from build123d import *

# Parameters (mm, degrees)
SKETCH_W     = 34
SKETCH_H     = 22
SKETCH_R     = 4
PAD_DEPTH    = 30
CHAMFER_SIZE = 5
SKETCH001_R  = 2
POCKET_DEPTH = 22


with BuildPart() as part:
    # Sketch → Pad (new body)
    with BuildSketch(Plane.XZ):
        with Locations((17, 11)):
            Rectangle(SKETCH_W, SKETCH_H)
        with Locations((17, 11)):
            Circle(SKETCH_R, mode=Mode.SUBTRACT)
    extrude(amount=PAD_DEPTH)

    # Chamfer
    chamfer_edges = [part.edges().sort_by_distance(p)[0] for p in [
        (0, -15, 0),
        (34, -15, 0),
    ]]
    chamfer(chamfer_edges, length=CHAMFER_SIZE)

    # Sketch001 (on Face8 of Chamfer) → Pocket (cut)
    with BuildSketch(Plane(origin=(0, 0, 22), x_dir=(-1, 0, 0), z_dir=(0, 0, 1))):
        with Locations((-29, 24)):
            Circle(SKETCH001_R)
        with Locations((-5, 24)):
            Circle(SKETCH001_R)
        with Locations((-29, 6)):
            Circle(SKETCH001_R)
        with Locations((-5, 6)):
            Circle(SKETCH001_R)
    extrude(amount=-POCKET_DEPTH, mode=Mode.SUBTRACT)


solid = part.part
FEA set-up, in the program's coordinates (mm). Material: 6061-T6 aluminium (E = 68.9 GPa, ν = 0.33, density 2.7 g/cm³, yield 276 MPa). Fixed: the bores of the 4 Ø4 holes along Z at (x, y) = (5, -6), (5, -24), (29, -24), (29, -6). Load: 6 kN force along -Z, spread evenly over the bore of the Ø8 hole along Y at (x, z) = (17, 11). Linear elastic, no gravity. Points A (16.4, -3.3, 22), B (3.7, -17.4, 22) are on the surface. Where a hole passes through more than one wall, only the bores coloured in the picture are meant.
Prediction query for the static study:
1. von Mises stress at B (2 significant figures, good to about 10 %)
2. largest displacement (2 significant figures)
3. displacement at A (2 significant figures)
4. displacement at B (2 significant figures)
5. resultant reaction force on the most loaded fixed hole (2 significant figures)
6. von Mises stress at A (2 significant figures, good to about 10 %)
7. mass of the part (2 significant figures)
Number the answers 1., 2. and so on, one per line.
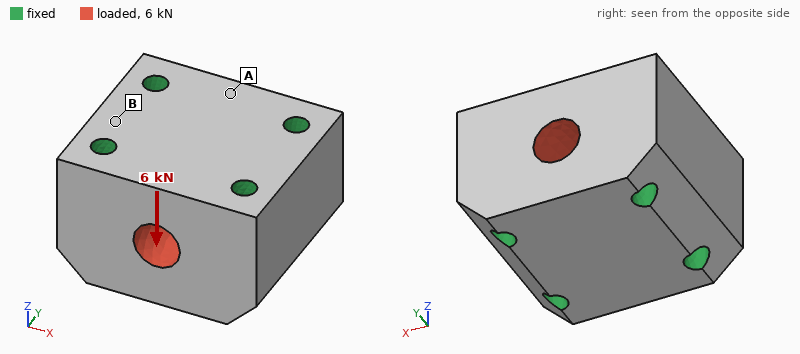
1. 3.1 MPa
2. 2.6 µm
3. 1.9 µm
4. 0.67 µm
5. 1.5 kN
6. 8.5 MPa
7. 52 g
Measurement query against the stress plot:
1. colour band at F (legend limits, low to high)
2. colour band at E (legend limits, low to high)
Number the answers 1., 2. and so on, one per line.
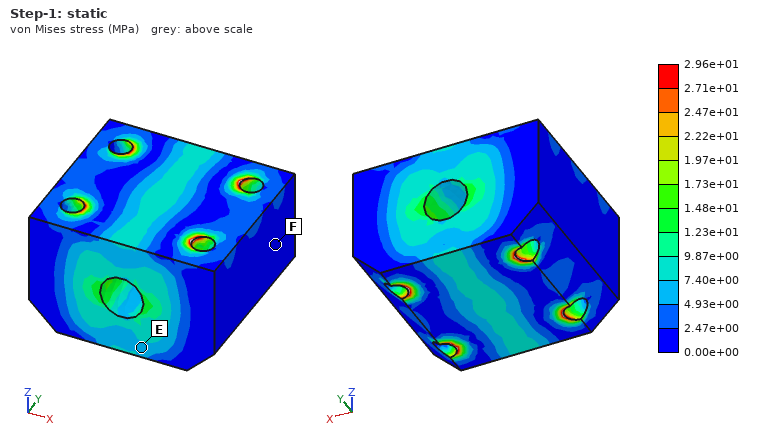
1. 0.00e+00 to 2.47e+00 MPa
2. 4.93e+00 to 7.40e+00 MPa
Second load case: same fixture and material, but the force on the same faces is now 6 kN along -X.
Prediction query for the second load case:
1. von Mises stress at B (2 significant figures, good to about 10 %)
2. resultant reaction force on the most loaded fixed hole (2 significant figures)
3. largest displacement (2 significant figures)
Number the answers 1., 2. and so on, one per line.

1. 1.8 MPa
2. 1.5 kN
3. 1.2 µm
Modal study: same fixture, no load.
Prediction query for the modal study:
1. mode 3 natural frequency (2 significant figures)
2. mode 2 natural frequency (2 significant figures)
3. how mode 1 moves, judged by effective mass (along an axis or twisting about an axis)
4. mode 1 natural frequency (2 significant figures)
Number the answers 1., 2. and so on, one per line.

1. 66 kHz
2. 63 kHz
3. along Z
4. 60 kHz
